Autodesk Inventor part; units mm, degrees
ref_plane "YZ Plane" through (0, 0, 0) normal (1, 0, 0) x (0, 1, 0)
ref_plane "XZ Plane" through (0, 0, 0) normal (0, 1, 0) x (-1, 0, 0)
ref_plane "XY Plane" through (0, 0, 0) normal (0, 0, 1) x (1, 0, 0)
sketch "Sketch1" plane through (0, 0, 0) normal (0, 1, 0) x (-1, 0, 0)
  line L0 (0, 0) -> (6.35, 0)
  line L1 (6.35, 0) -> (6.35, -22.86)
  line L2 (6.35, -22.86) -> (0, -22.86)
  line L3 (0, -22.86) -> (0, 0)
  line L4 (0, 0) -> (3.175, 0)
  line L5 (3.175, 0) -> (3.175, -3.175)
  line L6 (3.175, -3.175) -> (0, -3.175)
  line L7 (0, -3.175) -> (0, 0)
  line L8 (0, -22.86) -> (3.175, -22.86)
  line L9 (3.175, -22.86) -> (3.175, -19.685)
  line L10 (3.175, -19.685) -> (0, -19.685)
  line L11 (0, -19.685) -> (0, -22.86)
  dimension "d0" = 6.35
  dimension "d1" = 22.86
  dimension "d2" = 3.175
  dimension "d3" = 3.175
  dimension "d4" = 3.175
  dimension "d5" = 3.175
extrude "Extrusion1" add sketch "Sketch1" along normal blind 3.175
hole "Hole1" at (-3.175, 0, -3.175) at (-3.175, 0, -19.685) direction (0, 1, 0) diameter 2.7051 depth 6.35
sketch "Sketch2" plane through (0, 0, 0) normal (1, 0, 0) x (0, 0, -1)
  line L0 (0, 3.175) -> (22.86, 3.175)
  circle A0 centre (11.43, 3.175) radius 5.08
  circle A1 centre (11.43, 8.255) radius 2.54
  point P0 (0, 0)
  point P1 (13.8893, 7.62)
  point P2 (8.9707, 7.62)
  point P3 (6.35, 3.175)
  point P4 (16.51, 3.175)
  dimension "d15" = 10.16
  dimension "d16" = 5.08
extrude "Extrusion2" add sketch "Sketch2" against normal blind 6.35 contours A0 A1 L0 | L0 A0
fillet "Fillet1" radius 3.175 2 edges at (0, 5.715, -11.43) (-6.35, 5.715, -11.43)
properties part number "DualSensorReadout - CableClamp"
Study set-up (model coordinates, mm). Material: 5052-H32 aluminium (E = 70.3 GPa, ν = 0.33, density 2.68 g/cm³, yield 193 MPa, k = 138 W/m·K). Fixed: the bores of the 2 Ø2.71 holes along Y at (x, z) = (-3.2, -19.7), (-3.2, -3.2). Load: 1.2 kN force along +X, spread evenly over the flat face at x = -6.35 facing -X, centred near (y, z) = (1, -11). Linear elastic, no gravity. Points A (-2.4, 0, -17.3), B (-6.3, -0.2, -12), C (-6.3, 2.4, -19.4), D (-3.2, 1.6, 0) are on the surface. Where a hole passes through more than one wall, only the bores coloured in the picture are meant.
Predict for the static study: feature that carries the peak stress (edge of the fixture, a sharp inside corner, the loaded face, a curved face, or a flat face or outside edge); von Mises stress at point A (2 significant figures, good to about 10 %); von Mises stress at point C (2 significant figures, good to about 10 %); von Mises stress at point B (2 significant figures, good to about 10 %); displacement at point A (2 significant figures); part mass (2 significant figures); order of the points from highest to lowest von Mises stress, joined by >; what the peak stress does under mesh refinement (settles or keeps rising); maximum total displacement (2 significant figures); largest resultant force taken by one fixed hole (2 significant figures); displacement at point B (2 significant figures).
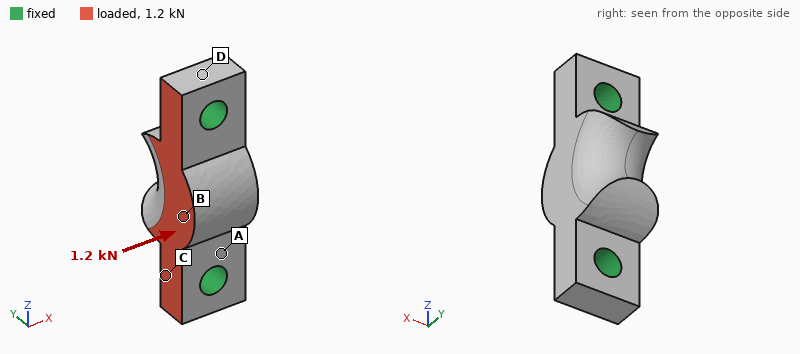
edge of the fixture
51 MPa
38 MPa
23 MPa
2.0 µm
1.8 g
A > C > B > D
keeps rising
8.2 µm
600 N
7.0 µm
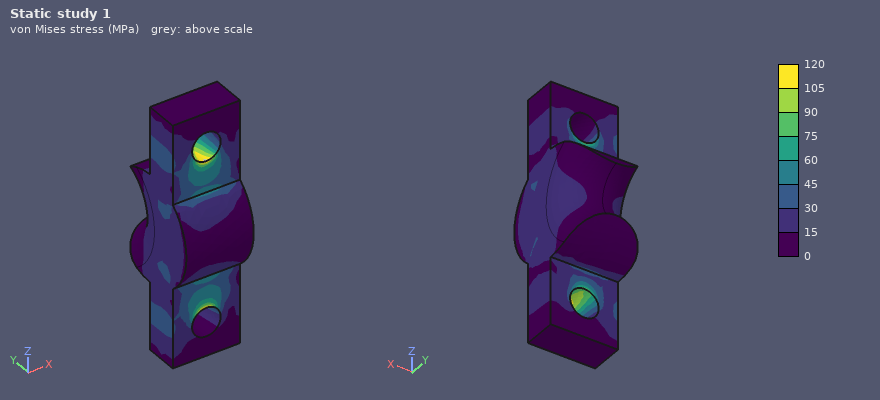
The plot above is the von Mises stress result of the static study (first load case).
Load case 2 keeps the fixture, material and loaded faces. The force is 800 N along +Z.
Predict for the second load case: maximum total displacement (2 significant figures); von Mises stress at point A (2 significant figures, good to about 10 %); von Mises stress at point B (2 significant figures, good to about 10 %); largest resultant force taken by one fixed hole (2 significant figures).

2.2 µm
13 MPa
18 MPa
420 N
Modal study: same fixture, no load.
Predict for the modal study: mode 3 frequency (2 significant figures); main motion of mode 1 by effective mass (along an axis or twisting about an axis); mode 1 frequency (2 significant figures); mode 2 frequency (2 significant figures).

57 kHz
along X
44 kHz
56 kHz
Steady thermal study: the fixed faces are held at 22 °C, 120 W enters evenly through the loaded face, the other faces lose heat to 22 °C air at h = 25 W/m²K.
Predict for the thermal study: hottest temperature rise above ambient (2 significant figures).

81 K
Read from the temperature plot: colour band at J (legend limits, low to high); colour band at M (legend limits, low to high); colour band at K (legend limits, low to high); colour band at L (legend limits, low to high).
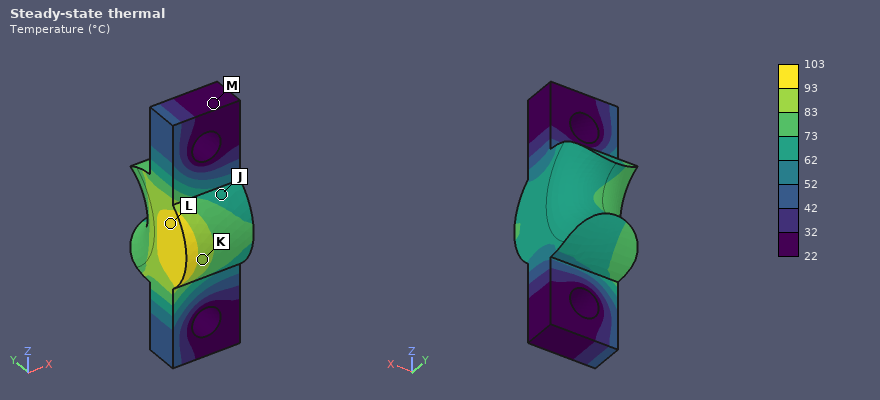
62 to 73 °C
22 to 32 °C
83 to 93 °C
93 to 103 °C
